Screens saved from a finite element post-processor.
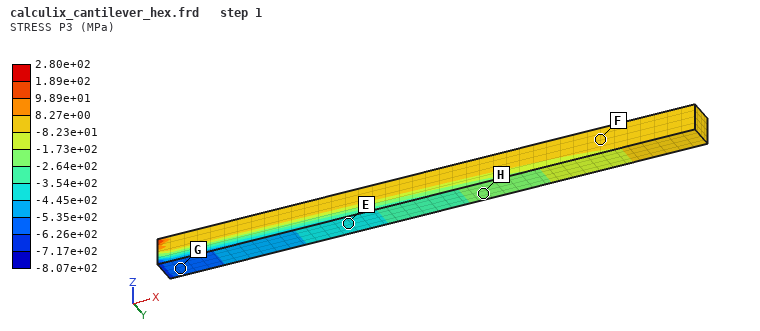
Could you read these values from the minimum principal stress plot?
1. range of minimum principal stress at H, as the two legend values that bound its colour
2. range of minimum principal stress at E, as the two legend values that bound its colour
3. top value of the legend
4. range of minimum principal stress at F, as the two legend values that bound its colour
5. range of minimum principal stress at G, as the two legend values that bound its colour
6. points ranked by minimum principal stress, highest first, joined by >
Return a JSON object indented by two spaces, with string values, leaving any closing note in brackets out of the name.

{
  "range of minimum principal stress at H, as the two legend values that bound its colour": "-2.64e+02 to -1.73e+02 MPa",
  "range of minimum principal stress at E, as the two legend values that bound its colour": "-4.45e+02 to -3.54e+02 MPa",
  "top value of the legend": "2.80e+02 MPa",
  "range of minimum principal stress at F, as the two legend values that bound its colour": "-8.23e+01 to 8.27e+00 MPa",
  "range of minimum principal stress at G, as the two legend values that bound its colour": "-6.26e+02 to -5.35e+02 MPa",
  "points ranked by minimum principal stress, highest first, joined by >": "F > H > E > G"
}
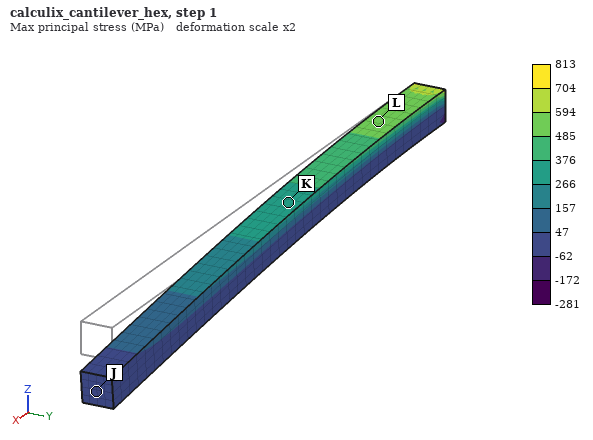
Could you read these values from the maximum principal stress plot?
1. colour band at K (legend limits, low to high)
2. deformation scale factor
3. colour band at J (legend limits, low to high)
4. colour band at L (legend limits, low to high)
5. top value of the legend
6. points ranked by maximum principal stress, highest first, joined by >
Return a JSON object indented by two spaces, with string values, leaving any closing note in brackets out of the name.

{
  "colour band at K": "266 to 376 MPa",
  "deformation scale factor": "2",
  "colour band at J": "-62 to 47 MPa",
  "colour band at L": "485 to 594 MPa",
  "top value of the legend": "813 MPa",
  "points ranked by maximum principal stress, highest first, joined by >": "L > K > J"
}
